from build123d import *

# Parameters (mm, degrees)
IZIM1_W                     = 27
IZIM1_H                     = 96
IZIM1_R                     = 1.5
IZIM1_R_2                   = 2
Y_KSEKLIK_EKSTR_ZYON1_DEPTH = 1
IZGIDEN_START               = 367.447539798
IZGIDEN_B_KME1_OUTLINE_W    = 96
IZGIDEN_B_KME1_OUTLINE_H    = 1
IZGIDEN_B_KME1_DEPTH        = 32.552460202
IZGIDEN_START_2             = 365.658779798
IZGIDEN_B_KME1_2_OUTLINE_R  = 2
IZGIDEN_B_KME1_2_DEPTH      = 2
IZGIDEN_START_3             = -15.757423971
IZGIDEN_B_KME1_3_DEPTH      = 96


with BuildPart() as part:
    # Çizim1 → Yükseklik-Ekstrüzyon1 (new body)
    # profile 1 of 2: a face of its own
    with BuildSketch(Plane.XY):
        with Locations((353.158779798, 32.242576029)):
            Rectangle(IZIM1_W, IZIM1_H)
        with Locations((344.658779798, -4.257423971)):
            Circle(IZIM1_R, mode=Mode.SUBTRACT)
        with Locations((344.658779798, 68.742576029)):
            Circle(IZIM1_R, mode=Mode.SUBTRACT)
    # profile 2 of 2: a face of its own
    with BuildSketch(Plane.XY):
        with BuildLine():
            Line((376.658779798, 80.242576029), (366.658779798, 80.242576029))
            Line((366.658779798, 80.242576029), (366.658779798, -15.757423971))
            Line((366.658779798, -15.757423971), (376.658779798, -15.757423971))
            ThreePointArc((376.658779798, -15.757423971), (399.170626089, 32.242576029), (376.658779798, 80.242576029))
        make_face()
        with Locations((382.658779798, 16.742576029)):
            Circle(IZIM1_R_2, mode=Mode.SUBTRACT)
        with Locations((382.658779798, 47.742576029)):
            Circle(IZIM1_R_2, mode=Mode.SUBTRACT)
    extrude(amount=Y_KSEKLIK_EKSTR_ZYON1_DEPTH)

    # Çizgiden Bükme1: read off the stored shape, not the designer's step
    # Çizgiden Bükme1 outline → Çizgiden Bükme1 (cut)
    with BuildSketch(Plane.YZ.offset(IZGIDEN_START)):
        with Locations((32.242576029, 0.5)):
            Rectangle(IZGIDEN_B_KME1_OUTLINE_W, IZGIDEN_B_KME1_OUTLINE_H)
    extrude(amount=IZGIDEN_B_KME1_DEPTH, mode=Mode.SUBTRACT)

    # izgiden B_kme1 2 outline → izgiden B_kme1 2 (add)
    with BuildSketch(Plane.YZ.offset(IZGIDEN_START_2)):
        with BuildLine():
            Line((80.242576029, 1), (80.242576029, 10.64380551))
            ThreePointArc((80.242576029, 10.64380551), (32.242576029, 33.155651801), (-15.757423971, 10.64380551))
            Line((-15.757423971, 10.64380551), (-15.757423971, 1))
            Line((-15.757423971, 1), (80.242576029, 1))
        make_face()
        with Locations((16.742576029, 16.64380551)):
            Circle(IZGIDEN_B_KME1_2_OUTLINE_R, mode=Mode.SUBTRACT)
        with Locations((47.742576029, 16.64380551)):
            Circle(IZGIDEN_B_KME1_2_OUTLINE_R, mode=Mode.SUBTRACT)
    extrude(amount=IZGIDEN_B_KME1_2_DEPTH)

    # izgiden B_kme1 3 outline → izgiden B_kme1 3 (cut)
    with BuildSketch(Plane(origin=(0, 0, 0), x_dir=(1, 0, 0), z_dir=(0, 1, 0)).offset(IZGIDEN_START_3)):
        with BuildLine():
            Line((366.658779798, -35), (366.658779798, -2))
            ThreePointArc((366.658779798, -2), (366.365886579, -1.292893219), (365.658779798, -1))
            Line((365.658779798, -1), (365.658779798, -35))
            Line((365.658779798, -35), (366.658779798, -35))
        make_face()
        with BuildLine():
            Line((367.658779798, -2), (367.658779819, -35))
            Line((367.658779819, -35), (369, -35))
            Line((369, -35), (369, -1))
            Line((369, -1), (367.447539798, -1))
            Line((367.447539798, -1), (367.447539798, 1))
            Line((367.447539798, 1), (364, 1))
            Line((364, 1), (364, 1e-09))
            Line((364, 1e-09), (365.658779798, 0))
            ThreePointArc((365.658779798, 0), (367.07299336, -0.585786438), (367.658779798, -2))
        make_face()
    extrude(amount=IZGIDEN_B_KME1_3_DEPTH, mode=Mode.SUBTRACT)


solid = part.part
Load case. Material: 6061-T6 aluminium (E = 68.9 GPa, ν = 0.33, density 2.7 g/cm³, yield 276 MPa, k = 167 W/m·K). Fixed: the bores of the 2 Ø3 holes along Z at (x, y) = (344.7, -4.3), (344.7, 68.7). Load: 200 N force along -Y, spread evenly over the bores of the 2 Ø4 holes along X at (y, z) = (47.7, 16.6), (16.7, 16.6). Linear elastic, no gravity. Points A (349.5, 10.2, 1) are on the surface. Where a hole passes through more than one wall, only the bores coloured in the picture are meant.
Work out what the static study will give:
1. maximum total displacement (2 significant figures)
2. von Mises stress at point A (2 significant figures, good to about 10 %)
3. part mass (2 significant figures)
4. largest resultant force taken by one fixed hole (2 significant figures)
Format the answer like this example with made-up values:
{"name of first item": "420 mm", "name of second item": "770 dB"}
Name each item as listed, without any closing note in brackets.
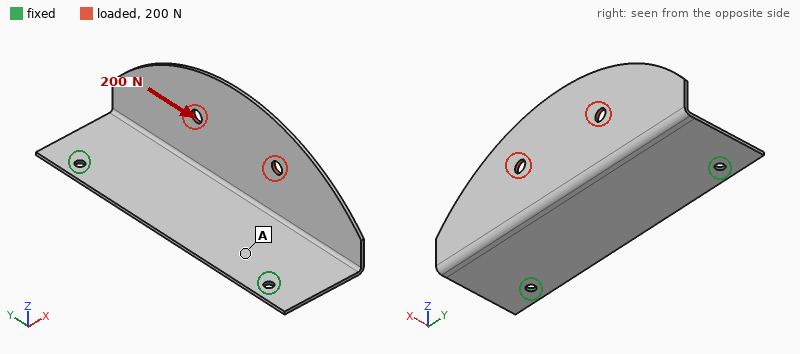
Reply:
{"maximum total displacement": "0.92 mm", "von Mises stress at point A": "38 MPa", "part mass": "14 g", "largest resultant force taken by one fixed hole": "120 N"}
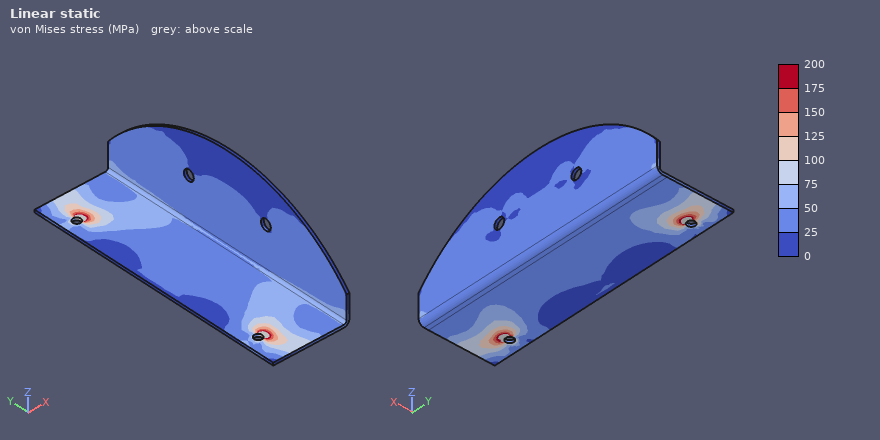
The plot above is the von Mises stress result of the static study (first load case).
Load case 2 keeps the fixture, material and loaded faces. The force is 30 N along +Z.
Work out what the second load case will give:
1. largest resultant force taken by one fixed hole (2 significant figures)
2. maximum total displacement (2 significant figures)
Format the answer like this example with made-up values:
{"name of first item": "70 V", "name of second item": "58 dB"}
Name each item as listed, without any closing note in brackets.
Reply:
{"largest resultant force taken by one fixed hole": "15 N", "maximum total displacement": "0.77 mm"}
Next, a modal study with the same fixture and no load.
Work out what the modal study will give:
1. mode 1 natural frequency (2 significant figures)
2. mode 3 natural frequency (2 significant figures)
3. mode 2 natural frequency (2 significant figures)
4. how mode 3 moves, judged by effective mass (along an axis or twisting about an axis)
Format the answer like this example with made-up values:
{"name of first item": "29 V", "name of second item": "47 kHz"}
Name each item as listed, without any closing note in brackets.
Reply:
{"mode 1 natural frequency": "370 Hz", "mode 3 natural frequency": "890 Hz", "mode 2 natural frequency": "760 Hz", "how mode 3 moves, judged by effective mass": "along Z"}
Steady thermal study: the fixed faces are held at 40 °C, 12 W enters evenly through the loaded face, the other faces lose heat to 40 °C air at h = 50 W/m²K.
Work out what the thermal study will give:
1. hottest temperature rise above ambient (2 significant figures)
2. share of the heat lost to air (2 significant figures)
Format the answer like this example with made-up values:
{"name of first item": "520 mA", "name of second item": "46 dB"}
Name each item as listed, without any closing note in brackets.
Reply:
{"hottest temperature rise above ambient": "33 K", "share of the heat lost to air": "62 %"}
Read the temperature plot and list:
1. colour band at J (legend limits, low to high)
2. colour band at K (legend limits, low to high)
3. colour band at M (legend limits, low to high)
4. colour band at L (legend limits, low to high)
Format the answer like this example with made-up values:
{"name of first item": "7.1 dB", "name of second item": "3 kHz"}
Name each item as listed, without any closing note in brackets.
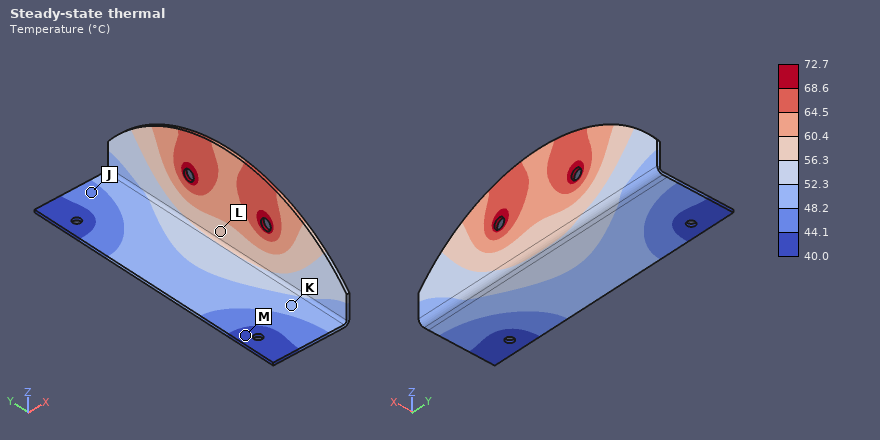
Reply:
{"colour band at J": "44.1 to 48.2 °C", "colour band at K": "48.2 to 52.3 °C", "colour band at M": "40.0 to 44.1 °C", "colour band at L": "56.3 to 60.4 °C"}
